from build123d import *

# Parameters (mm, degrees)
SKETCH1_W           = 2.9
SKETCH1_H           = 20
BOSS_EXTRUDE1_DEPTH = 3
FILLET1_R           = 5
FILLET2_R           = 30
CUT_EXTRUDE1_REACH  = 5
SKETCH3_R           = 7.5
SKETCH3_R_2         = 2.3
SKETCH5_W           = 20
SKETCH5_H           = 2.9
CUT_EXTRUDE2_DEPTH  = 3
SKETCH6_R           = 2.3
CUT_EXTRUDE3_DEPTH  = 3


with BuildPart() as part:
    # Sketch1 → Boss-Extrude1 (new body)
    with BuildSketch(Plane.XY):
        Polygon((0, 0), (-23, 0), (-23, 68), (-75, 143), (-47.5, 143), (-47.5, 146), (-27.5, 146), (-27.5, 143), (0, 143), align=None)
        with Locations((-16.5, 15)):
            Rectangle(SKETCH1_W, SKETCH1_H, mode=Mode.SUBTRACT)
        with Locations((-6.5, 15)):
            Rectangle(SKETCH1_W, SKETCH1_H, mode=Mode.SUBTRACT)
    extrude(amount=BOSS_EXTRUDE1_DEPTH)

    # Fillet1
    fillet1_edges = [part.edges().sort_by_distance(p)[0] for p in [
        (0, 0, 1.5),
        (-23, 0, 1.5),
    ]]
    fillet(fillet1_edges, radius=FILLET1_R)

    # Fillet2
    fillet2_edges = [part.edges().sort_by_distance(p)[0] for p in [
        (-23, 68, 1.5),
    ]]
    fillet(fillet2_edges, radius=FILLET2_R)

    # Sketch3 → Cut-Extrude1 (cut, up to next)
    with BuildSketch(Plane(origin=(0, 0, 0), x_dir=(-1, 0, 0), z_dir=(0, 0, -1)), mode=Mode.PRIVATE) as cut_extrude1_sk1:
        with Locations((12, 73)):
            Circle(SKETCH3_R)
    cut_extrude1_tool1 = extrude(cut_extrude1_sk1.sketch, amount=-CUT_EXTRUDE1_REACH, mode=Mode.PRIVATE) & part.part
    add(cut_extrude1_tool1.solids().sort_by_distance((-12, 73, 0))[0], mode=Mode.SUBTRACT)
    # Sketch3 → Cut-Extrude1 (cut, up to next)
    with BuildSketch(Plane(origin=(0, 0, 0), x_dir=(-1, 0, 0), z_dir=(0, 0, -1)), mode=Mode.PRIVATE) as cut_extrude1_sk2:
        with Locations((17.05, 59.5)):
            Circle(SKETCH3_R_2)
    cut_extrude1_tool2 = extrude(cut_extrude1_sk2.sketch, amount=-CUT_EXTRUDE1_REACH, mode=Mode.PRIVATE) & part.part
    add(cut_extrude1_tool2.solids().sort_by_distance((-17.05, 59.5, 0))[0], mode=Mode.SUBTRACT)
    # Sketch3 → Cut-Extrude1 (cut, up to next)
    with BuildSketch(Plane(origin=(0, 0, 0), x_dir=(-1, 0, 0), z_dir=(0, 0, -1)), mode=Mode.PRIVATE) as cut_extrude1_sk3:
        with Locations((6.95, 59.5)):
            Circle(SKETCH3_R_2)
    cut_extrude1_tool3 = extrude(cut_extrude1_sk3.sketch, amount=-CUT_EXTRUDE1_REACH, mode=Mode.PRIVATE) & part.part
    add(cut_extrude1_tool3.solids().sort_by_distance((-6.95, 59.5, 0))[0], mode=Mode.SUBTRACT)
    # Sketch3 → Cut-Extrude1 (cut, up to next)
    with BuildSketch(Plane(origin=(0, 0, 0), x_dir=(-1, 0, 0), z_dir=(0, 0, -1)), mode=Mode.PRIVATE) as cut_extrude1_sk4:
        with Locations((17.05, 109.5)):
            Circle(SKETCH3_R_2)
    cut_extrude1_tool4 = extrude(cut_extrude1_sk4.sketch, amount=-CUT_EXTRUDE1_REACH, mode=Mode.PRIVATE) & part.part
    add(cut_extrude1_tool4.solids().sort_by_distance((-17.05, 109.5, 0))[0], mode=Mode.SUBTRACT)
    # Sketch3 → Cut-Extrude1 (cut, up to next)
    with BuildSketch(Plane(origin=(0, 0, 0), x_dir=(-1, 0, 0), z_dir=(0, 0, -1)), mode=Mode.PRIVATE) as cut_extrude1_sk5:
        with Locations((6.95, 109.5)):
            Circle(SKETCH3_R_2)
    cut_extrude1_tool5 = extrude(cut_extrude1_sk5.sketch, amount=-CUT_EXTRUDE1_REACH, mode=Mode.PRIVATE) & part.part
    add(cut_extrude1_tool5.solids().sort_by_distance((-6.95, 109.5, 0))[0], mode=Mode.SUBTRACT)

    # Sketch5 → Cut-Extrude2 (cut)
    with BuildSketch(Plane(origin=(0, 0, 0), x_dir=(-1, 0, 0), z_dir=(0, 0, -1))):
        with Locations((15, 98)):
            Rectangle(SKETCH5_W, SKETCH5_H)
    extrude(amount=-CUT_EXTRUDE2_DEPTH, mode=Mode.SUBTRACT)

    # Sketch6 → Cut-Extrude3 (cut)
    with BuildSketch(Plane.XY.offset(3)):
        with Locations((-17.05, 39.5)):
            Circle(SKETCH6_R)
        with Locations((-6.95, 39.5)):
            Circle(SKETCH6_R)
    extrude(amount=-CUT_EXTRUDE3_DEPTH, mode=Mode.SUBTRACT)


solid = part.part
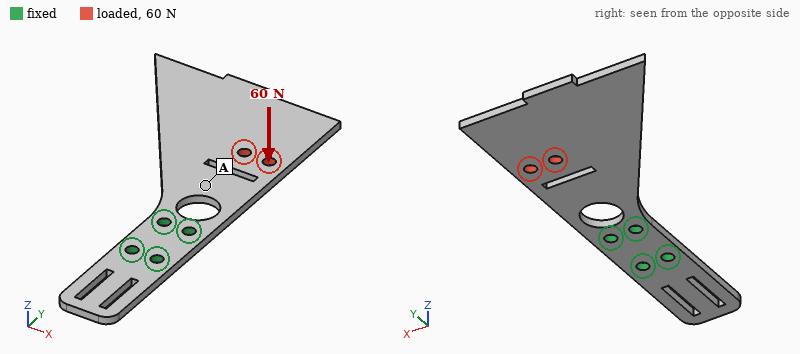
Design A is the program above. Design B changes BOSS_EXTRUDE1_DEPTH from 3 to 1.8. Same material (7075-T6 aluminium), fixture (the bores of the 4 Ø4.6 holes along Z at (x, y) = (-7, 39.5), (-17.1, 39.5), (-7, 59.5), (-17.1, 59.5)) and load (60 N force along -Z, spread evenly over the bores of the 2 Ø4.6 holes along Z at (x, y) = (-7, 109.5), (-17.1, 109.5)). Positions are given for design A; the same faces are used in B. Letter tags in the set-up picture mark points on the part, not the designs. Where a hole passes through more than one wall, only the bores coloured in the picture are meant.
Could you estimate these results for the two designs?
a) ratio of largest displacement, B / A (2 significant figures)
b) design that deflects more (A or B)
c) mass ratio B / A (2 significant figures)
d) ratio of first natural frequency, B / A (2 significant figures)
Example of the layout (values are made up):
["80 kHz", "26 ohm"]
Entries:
["4.5", "B", "0.60", "0.61"]
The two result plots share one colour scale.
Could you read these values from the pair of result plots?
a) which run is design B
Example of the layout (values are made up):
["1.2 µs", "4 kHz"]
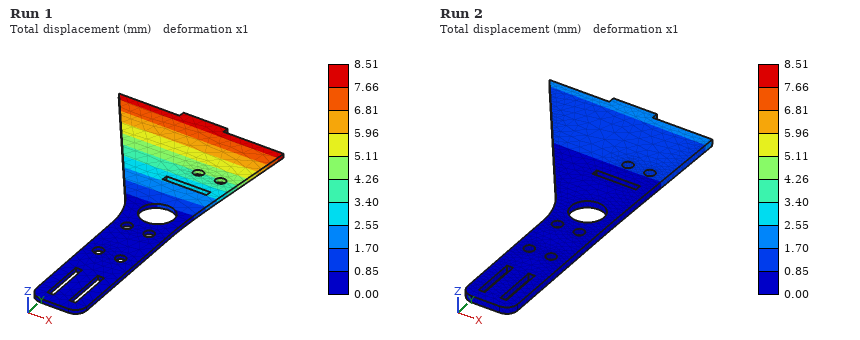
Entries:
["Run 1"]
